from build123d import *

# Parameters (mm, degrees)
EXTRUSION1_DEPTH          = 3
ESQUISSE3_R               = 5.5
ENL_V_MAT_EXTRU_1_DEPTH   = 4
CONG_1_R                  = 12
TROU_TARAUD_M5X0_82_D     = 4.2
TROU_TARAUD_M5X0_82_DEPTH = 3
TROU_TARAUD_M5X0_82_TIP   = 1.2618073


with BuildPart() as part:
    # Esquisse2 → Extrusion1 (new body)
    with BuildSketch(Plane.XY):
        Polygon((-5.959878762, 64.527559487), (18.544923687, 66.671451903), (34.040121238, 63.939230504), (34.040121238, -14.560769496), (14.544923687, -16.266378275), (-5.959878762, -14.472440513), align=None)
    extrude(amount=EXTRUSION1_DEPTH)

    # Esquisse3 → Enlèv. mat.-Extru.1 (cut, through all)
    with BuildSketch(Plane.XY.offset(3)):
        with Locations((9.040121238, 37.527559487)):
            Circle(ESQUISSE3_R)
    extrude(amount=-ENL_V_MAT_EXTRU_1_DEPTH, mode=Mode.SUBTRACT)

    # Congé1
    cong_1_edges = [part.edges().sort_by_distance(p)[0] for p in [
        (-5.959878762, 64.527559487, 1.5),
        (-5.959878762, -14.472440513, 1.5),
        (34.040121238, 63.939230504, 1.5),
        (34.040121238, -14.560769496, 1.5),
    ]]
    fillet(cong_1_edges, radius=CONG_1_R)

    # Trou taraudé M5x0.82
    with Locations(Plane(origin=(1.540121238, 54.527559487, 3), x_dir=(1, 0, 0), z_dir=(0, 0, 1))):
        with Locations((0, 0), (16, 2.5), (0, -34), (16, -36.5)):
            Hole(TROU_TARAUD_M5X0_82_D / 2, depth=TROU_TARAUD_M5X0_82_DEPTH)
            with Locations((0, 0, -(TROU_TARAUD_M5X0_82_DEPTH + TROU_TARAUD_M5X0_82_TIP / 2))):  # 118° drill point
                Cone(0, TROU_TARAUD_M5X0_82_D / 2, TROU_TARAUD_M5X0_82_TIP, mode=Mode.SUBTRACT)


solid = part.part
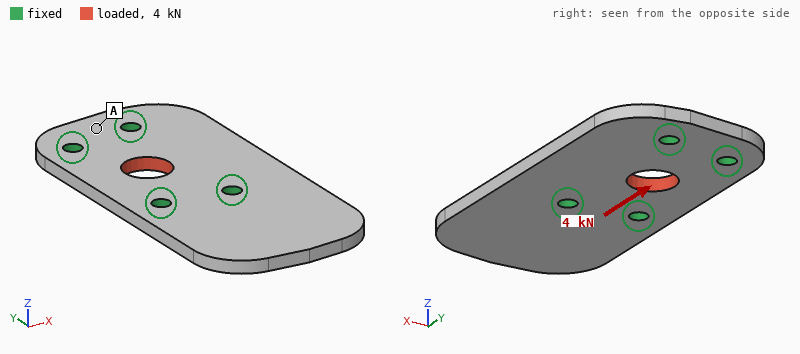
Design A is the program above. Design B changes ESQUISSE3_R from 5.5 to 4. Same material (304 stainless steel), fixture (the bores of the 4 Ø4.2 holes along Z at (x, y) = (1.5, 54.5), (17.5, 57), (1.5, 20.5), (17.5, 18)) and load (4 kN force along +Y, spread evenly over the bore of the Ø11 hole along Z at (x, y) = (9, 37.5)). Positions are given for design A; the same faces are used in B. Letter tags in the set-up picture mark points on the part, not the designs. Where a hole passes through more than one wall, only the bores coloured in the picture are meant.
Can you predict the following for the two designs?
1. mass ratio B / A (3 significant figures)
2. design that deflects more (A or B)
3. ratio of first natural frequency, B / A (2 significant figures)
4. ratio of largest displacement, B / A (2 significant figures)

1.01
B
1.0
1.2
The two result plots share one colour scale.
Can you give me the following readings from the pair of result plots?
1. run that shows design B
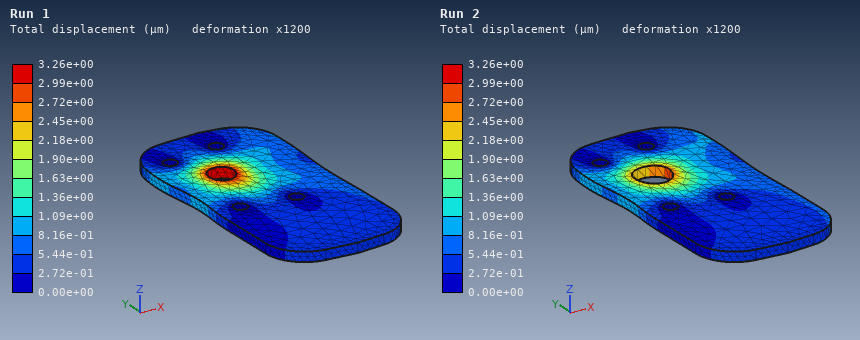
Run 1
